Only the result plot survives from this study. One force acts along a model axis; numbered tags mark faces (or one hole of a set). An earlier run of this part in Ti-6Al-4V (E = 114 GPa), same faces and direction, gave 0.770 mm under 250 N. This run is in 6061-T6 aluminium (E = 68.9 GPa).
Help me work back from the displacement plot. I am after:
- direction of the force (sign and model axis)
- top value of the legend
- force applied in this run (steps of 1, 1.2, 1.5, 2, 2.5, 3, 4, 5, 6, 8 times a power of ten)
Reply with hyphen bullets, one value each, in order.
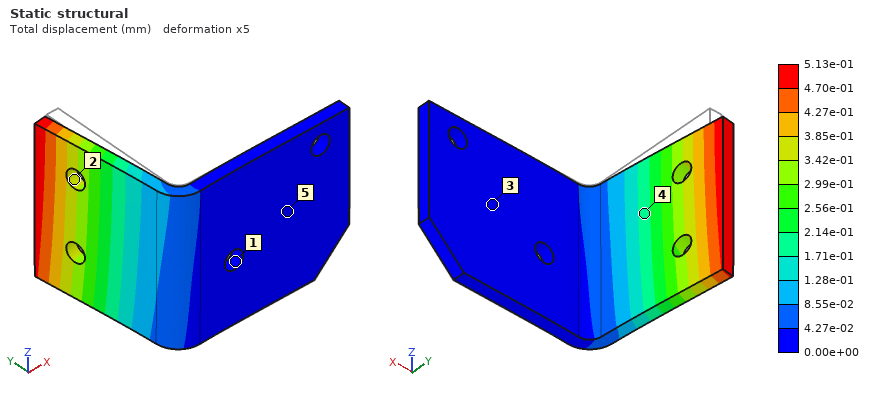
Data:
- -X
- 5.13e-01 mm
- 100 N
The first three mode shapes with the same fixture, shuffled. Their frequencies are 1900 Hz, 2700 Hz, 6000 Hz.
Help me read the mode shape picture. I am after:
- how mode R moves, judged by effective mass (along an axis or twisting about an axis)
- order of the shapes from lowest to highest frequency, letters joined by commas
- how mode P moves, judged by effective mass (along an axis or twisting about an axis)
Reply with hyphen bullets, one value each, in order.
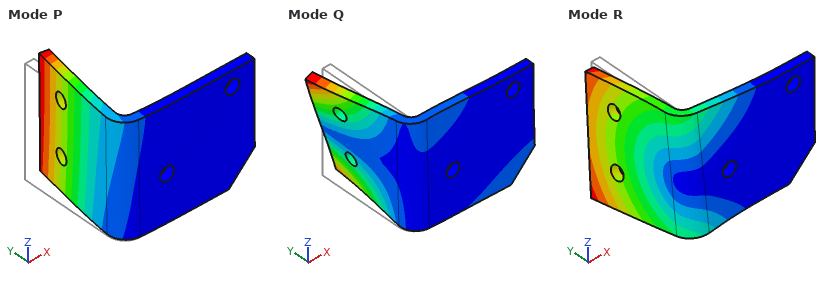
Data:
- along Z
- P, R, Q
- along X
